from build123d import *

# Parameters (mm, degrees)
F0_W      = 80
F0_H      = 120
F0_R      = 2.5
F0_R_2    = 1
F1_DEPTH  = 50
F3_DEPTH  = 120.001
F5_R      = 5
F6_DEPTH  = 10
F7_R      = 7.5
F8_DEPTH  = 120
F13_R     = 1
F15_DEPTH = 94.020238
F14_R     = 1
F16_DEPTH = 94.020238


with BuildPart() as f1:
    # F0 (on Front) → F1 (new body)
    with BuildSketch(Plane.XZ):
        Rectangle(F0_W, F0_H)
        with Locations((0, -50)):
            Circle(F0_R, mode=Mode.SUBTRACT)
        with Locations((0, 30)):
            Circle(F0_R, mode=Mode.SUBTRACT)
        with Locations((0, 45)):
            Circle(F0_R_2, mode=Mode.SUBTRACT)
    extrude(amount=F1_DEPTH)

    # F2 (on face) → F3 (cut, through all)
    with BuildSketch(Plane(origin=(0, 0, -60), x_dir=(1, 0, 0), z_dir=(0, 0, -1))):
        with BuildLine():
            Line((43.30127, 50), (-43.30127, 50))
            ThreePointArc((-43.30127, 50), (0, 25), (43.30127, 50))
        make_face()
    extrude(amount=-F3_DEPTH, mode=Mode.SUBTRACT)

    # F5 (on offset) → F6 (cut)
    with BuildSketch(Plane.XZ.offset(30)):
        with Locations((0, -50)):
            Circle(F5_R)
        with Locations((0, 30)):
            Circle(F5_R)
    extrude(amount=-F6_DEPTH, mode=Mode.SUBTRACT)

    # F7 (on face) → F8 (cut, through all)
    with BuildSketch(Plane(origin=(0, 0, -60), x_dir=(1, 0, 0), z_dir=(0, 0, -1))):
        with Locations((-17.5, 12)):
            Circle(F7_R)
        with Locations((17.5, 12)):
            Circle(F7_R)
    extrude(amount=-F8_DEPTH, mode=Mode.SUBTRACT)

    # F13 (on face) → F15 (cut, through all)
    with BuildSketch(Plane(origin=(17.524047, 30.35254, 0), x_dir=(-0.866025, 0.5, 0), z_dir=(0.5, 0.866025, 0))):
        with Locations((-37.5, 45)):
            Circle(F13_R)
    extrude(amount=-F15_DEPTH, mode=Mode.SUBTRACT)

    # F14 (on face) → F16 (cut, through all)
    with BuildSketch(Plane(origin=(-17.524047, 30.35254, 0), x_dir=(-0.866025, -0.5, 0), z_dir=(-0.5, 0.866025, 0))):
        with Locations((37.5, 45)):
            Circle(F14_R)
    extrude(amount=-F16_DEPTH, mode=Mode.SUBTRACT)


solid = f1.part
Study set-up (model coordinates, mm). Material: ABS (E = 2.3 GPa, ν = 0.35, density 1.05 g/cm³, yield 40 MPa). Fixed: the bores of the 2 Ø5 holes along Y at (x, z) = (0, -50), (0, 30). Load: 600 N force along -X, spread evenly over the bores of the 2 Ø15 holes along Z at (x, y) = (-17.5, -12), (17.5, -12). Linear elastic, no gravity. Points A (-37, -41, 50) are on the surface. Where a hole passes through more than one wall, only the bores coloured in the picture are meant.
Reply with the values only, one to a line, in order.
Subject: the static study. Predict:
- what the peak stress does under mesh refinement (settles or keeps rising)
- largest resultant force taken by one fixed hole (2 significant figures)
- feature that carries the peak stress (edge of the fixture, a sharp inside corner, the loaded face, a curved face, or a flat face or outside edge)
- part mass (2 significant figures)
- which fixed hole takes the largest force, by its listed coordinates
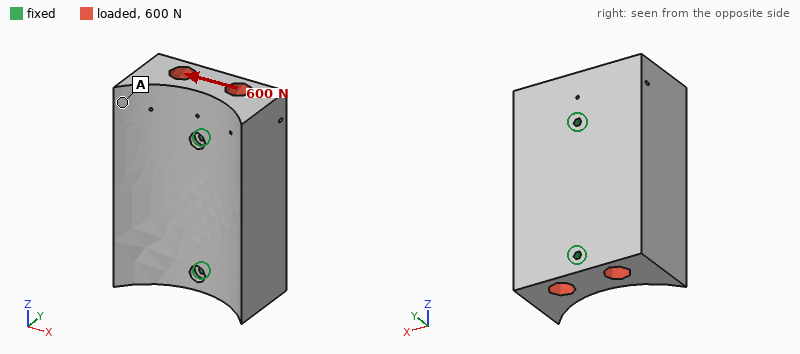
keeps rising
370 N
edge of the fixture
270 g
(0, 30)
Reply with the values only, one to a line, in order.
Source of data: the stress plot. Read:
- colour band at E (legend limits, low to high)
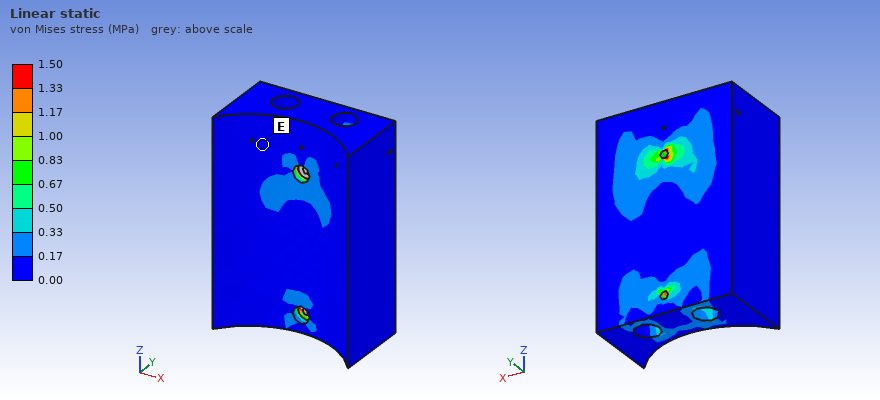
0.00 to 0.17 MPa
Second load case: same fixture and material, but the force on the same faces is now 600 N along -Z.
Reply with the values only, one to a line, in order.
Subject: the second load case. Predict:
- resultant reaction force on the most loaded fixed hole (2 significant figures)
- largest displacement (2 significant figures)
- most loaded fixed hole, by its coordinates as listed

350 N
6.9 µm
(0, 30)
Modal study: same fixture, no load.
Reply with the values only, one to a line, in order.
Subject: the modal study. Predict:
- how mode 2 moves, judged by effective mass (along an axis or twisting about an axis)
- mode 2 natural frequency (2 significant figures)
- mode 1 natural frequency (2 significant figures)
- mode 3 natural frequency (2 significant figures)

along Y
1600 Hz
900 Hz
2000 Hz
